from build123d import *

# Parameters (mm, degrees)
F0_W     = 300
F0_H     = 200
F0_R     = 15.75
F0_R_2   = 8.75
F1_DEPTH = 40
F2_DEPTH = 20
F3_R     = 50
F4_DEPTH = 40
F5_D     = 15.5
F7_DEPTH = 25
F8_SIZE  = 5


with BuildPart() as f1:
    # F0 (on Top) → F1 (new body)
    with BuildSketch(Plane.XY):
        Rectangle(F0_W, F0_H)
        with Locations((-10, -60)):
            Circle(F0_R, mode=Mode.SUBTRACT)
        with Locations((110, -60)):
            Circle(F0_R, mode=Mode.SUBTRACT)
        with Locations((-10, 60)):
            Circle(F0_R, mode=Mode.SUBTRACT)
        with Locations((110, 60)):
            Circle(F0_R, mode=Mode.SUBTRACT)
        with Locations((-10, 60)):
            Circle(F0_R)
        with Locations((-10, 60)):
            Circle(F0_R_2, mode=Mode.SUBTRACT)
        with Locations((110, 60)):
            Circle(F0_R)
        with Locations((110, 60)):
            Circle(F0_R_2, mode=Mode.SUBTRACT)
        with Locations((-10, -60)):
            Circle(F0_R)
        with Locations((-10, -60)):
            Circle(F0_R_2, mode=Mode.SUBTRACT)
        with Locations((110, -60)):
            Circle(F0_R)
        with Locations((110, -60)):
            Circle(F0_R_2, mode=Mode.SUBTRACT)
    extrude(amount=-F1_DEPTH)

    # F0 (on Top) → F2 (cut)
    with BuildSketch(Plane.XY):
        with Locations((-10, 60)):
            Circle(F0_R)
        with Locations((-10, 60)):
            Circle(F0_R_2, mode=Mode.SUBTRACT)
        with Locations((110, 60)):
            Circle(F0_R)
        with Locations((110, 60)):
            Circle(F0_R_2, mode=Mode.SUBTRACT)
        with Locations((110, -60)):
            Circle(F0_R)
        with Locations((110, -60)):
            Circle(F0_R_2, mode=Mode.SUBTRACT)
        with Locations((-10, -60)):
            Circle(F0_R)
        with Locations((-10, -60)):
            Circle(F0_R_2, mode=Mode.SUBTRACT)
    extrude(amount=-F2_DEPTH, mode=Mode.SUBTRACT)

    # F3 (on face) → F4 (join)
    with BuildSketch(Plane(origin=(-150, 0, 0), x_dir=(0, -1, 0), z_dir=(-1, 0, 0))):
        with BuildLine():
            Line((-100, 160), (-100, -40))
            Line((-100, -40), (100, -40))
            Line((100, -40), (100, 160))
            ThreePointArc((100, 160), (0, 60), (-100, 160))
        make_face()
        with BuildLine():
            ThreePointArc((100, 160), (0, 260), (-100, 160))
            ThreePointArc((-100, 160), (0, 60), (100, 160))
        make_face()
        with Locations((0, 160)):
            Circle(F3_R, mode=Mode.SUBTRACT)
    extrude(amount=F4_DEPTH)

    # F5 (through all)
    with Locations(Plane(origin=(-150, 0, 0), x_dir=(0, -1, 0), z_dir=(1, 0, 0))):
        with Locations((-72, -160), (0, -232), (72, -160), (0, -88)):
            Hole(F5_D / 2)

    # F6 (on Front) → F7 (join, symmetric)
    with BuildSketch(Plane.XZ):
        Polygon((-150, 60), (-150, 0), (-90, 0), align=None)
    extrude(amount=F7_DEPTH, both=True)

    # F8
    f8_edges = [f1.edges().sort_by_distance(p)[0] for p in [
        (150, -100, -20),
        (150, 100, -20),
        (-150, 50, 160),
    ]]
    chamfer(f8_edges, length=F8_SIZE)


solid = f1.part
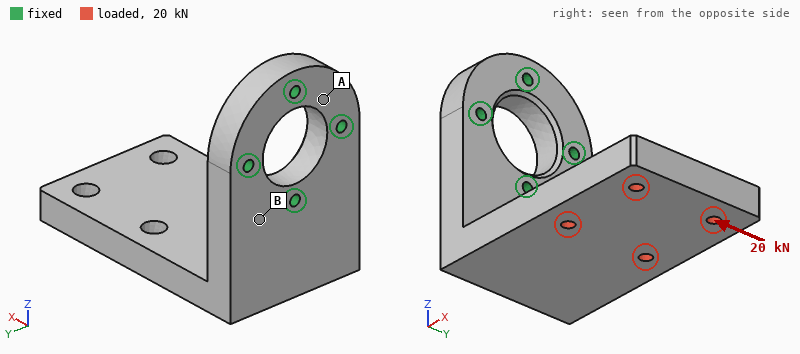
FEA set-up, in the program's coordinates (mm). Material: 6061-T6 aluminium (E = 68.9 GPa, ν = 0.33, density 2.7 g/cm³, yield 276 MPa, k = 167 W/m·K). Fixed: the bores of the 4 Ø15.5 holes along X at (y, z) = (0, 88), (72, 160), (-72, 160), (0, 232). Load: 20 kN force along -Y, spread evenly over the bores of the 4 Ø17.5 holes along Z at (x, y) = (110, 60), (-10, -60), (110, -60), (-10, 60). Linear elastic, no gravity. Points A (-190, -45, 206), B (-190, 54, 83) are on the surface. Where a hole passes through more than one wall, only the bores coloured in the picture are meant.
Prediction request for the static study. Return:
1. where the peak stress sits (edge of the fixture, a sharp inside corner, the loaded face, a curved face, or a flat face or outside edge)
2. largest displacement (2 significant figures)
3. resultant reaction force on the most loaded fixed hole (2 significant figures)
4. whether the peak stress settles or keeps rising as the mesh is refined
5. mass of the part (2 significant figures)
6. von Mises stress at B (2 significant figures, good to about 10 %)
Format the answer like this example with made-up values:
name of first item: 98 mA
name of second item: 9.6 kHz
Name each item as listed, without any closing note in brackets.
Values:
where the peak stress sits: edge of the fixture
largest displacement: 1.4 mm
resultant reaction force on the most loaded fixed hole: 20 kN
whether the peak stress settles or keeps rising as the mesh is refined: keeps rising
mass of the part: 12 kg
von Mises stress at B: 35 MPa
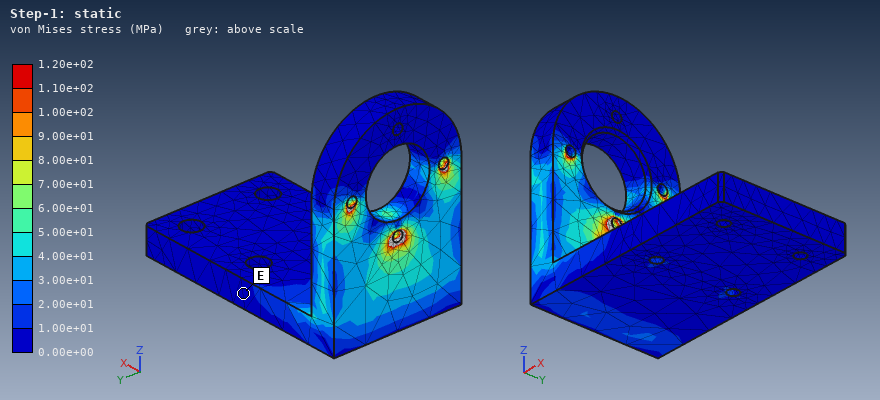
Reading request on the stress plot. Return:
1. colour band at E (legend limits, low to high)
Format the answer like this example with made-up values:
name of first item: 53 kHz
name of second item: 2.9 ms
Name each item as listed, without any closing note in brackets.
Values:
colour band at E: 0.00e+00 to 1.00e+01 MPa
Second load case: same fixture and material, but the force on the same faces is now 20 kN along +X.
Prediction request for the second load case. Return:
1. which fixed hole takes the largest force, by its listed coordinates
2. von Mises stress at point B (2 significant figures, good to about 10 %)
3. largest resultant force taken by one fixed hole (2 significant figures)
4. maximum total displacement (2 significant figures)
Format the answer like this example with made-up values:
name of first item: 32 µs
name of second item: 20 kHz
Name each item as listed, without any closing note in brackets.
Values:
which fixed hole takes the largest force, by its listed coordinates: (0, 88)
von Mises stress at point B: 24 MPa
largest resultant force taken by one fixed hole: 31 kN
maximum total displacement: 0.83 mm
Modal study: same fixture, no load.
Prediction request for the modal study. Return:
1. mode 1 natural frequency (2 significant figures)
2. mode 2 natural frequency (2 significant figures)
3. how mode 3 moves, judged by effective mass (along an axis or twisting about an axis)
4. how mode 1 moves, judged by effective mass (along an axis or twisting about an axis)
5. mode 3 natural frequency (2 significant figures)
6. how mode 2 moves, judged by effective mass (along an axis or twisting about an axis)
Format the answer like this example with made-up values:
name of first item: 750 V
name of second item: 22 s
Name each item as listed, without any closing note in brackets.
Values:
mode 1 natural frequency: 240 Hz
mode 2 natural frequency: 330 Hz
how mode 3 moves, judged by effective mass: along X
how mode 1 moves, judged by effective mass: along Z
mode 3 natural frequency: 850 Hz
how mode 2 moves, judged by effective mass: along Y
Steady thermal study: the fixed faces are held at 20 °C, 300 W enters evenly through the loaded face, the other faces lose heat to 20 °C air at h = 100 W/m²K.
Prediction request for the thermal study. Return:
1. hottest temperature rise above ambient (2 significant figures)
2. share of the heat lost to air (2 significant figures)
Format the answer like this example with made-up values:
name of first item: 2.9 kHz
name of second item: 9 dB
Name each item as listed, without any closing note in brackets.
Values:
hottest temperature rise above ambient: 23 K
share of the heat lost to air: 83 %
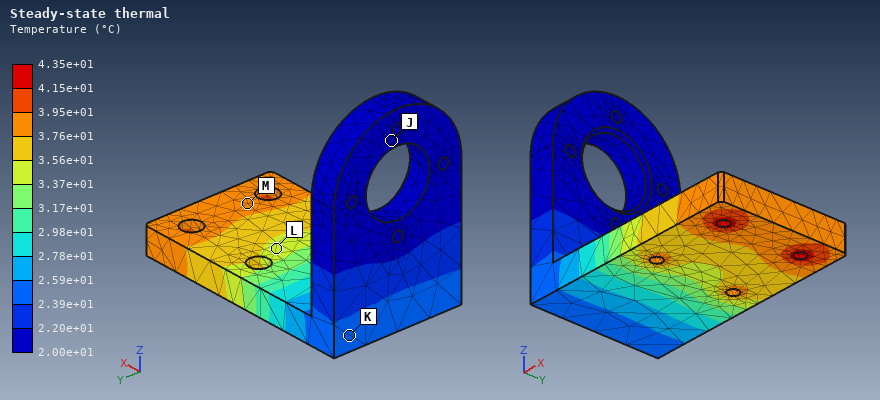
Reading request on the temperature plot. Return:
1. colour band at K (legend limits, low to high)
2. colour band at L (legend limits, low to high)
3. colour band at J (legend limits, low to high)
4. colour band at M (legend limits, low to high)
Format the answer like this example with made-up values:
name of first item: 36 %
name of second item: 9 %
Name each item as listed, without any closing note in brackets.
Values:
colour band at K: 2.39e+01 to 2.59e+01 °C
colour band at L: 3.37e+01 to 3.56e+01 °C
colour band at J: 2.00e+01 to 2.20e+01 °C
colour band at M: 3.76e+01 to 3.95e+01 °C
